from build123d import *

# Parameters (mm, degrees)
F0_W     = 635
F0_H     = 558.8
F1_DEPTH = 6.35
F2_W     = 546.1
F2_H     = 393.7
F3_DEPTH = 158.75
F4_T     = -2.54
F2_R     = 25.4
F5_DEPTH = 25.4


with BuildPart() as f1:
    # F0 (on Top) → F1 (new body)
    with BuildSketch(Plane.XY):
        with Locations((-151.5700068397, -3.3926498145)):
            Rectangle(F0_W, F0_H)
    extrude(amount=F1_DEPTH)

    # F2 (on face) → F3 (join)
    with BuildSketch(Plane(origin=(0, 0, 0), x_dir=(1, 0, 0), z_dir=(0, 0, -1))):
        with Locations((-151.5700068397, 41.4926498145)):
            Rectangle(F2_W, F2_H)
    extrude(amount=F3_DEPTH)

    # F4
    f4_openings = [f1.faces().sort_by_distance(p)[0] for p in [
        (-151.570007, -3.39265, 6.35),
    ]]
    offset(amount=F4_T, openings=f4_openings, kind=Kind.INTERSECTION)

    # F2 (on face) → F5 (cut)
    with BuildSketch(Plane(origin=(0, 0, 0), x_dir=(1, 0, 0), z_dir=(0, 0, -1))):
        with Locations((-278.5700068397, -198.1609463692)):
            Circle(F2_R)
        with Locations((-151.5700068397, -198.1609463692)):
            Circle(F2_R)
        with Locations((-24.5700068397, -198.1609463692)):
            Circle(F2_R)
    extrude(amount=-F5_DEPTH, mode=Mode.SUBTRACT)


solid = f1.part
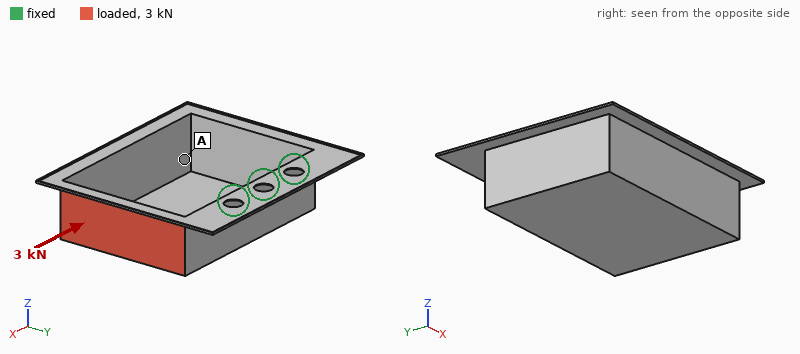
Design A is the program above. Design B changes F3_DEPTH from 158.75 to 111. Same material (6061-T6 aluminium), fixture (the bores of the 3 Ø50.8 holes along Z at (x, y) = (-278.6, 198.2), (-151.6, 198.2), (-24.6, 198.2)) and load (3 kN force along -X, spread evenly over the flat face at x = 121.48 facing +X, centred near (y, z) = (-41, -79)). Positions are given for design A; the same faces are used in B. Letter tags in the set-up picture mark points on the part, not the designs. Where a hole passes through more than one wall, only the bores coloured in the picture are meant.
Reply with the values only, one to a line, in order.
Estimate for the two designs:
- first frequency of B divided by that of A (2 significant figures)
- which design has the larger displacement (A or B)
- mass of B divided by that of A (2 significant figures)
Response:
1.2
B
0.86
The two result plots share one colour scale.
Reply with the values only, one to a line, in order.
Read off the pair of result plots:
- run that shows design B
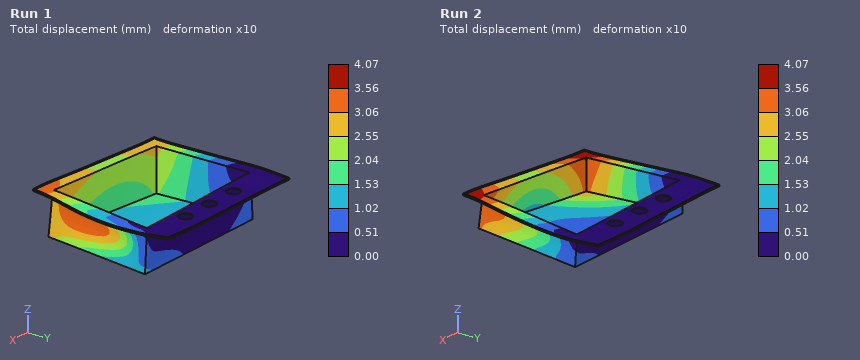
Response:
Run 2
